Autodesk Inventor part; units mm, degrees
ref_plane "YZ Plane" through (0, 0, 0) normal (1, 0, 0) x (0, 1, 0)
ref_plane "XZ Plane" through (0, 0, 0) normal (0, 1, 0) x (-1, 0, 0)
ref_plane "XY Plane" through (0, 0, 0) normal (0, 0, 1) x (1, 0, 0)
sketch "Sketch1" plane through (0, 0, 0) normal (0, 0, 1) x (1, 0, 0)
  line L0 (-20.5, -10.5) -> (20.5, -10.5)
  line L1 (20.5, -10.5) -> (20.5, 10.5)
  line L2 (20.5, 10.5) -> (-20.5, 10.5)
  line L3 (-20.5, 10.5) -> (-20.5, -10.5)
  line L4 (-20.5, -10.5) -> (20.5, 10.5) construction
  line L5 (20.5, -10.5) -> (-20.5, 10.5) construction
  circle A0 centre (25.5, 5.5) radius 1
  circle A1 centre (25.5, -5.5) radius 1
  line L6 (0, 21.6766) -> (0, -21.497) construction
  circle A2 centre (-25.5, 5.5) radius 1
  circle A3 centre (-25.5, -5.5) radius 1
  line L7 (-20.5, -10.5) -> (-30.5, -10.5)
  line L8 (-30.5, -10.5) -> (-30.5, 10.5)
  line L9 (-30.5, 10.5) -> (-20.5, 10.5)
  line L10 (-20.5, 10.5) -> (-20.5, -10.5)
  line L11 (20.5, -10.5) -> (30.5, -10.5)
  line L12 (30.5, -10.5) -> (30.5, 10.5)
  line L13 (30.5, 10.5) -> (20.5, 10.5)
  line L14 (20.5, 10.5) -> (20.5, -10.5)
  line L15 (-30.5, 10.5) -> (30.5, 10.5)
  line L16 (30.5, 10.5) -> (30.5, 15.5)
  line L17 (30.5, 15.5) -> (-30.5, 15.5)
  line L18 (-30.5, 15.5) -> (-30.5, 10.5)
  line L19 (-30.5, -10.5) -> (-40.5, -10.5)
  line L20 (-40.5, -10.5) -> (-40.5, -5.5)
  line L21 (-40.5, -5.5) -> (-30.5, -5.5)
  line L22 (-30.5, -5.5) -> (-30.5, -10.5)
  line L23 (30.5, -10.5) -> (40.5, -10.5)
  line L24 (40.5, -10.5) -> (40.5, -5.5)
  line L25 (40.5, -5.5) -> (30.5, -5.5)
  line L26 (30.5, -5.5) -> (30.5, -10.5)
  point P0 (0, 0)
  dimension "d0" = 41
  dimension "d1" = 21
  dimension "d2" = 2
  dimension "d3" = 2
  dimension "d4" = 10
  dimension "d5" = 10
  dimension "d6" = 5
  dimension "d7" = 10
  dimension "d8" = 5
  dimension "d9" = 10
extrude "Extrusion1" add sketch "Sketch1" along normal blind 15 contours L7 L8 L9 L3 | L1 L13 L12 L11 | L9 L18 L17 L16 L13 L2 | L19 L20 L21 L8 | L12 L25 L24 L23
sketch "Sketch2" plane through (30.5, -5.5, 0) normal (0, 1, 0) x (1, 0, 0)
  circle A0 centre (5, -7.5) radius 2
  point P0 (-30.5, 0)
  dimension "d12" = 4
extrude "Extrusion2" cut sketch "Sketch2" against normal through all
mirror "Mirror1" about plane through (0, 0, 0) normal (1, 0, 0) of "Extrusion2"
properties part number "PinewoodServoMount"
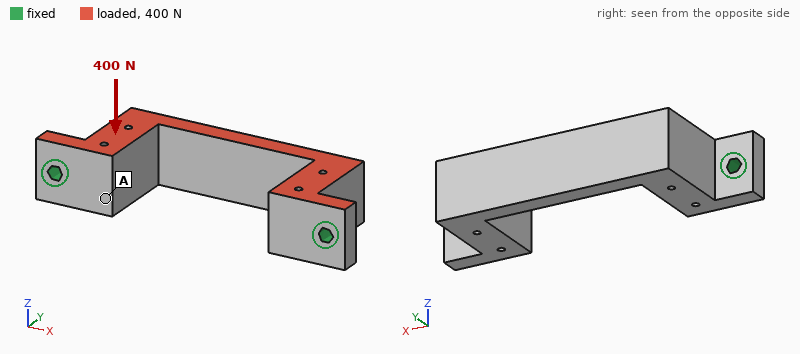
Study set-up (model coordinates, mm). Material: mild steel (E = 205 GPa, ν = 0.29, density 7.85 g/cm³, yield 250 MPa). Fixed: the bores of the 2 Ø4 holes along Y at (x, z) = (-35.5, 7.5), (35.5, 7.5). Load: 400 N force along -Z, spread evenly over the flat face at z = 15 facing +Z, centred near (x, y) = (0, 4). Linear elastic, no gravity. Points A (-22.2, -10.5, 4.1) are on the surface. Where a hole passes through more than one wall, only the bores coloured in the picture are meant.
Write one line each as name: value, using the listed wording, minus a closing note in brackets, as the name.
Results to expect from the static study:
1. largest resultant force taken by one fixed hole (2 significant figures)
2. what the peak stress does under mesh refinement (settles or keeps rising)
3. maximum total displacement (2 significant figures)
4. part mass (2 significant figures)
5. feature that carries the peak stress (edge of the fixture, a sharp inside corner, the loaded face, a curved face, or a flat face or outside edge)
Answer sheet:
largest resultant force taken by one fixed hole: 200 N
what the peak stress does under mesh refinement: keeps rising
maximum total displacement: 9.9 µm
part mass: 95 g
feature that carries the peak stress: edge of the fixture
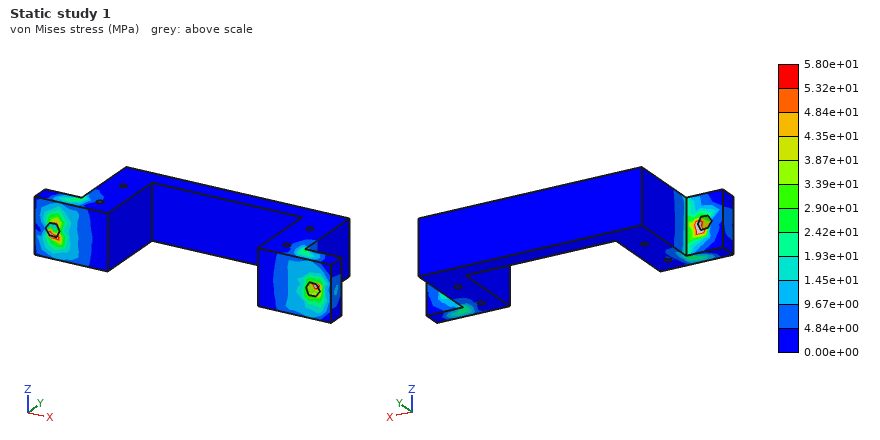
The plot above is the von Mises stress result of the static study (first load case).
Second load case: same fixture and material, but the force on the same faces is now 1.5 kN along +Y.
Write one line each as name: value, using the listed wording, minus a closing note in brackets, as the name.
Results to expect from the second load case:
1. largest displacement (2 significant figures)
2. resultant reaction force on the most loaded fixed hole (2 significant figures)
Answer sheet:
largest displacement: 23 µm
resultant reaction force on the most loaded fixed hole: 800 N
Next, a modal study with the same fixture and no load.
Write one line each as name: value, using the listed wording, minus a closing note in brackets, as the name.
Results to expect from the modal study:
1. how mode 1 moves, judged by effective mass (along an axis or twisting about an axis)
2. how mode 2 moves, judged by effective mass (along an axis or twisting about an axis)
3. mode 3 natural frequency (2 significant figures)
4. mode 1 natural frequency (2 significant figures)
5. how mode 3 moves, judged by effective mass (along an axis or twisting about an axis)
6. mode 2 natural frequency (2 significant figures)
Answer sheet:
how mode 1 moves, judged by effective mass: along Z
how mode 2 moves, judged by effective mass: along X
mode 3 natural frequency: 7000 Hz
mode 1 natural frequency: 3800 Hz
how mode 3 moves, judged by effective mass: twisting about Y
mode 2 natural frequency: 4800 Hz
